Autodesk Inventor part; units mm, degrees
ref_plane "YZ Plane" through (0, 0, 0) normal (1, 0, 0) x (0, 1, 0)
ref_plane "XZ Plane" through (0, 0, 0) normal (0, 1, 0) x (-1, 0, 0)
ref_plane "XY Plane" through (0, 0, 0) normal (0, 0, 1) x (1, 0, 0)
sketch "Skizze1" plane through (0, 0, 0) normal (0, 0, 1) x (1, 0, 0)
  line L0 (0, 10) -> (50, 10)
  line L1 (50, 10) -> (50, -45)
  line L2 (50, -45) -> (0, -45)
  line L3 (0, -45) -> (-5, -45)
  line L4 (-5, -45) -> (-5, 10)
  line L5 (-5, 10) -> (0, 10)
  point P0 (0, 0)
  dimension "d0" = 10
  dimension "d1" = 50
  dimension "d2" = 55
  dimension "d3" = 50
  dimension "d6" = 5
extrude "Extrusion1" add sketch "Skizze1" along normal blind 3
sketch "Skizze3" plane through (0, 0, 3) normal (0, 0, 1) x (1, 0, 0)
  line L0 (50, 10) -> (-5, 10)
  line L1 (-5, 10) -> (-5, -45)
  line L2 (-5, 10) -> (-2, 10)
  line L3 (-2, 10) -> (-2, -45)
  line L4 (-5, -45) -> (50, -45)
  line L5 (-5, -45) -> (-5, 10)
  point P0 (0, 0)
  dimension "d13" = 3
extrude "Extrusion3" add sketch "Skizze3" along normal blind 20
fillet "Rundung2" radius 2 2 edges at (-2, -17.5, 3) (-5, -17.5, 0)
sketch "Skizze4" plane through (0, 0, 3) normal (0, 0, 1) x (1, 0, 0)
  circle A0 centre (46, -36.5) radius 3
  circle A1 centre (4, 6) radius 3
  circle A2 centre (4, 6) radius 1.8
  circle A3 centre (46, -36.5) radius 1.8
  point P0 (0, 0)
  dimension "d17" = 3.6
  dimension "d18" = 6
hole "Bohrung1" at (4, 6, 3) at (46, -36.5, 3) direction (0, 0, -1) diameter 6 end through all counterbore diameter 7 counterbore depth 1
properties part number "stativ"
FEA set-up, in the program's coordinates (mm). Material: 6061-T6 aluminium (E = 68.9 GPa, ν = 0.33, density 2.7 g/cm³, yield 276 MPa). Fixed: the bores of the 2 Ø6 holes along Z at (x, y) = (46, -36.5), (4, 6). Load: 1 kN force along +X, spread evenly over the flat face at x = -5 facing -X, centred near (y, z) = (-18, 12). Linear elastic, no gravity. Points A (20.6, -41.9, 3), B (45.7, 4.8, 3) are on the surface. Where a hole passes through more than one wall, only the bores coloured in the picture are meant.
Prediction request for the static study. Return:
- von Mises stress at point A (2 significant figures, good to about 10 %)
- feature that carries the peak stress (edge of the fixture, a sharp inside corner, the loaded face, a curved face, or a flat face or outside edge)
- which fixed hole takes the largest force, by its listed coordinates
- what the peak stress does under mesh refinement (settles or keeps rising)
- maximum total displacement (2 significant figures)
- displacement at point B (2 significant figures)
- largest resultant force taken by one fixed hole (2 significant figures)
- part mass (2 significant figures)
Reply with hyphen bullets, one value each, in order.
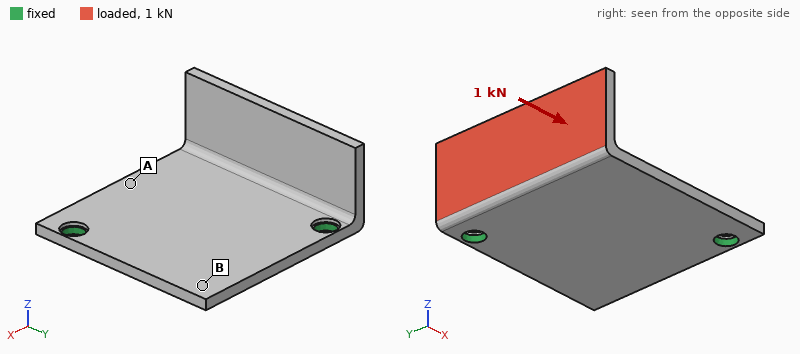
- 60 MPa
- edge of the fixture
- (46, -36.5)
- keeps rising
- 0.73 mm
- 0.13 mm
- 580 N
- 33 g
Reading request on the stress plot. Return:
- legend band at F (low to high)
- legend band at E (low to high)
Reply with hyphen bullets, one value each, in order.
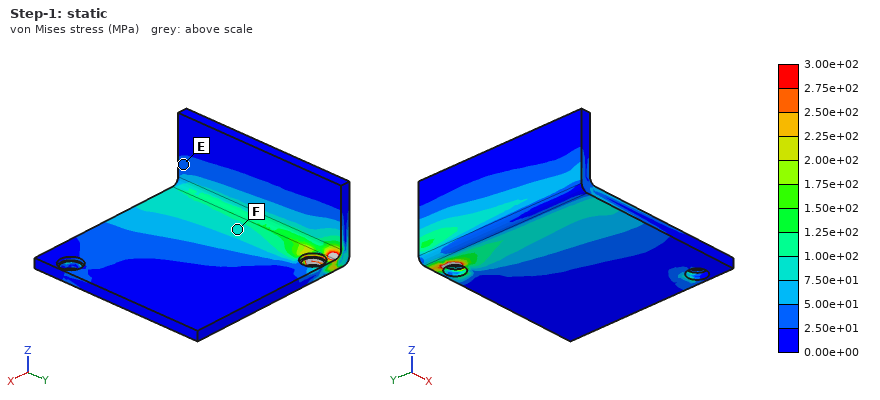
- 7.50e+01 to 1.00e+02 MPa
- 2.50e+01 to 5.00e+01 MPa
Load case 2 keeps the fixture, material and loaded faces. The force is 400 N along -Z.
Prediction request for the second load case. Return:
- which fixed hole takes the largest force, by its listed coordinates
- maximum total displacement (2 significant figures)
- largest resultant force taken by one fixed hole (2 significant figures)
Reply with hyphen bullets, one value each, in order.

- (4, 6)
- 0.59 mm
- 370 N
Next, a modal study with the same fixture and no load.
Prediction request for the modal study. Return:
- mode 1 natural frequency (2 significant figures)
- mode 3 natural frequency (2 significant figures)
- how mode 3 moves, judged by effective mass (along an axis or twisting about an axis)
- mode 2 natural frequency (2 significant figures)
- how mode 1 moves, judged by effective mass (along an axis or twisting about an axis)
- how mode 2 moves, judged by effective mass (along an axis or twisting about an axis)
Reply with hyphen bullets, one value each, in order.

- 1300 Hz
- 3100 Hz
- along X
- 2300 Hz
- along Z
- along Z
